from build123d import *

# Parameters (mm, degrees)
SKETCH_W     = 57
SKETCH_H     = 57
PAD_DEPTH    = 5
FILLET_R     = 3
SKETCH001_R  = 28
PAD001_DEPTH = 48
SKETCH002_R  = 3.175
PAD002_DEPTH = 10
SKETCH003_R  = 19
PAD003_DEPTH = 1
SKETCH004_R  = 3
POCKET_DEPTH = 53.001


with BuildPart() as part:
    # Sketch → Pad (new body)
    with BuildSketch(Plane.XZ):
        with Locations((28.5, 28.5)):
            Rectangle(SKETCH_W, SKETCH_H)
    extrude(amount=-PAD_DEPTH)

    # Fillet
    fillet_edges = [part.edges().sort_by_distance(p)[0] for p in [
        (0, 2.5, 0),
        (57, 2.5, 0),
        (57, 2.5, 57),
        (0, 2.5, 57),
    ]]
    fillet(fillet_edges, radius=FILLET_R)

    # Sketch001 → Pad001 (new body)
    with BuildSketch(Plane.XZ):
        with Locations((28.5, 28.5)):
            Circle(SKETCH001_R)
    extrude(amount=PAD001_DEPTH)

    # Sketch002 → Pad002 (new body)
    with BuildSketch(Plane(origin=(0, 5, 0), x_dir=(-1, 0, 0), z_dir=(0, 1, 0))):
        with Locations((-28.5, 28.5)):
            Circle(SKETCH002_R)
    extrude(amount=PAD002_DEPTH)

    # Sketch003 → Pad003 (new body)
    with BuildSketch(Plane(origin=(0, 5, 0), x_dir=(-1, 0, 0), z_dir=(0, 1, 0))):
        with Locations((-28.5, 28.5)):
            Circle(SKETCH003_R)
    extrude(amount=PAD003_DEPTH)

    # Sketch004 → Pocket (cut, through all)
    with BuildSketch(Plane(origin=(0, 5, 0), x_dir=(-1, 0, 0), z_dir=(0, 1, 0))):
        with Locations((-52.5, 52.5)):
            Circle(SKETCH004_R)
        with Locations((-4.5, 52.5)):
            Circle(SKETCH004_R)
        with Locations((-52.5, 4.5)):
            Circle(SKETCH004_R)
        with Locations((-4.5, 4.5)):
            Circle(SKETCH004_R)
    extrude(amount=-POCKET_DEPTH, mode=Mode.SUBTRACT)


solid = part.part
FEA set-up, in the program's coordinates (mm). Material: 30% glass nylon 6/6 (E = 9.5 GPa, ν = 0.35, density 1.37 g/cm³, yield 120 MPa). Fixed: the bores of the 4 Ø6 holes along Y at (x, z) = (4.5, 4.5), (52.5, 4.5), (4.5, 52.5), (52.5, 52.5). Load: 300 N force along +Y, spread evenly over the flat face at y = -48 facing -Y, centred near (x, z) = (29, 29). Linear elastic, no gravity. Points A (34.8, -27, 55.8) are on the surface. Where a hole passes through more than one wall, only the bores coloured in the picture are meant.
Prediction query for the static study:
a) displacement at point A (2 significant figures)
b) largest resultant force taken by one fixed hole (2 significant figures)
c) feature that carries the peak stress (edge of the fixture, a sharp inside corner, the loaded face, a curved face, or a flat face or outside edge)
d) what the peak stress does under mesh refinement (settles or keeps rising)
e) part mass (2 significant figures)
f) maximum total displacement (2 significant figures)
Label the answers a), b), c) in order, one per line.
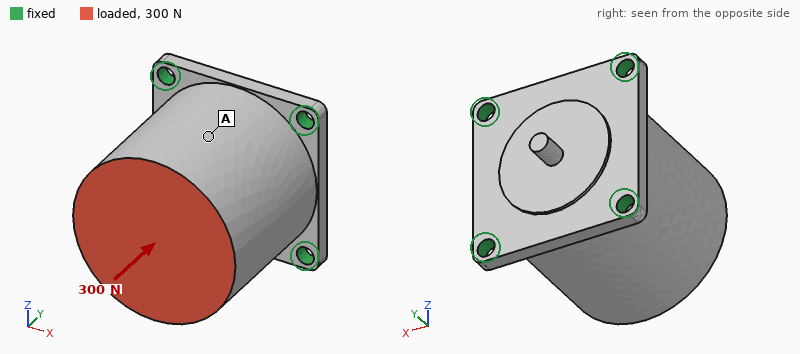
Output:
a) 4.1 µm
b) 82 N
c) edge of the fixture
d) keeps rising
e) 190 g
f) 4.3 µm
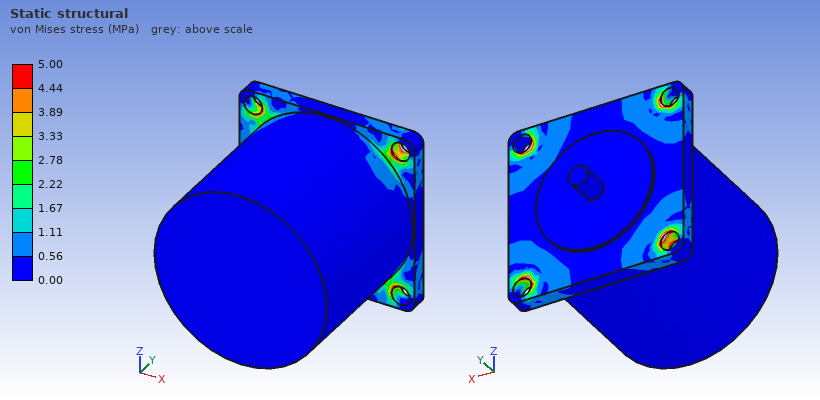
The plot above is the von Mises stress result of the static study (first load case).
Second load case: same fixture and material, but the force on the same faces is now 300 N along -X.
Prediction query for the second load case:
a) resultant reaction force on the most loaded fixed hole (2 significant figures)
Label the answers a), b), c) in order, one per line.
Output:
a) 200 N
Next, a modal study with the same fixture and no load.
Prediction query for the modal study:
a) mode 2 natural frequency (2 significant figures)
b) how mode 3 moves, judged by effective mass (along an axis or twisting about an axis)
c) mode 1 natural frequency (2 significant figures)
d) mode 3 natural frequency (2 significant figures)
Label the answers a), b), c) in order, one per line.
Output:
a) 2100 Hz
b) along Y
c) 2100 Hz
d) 3300 Hz
